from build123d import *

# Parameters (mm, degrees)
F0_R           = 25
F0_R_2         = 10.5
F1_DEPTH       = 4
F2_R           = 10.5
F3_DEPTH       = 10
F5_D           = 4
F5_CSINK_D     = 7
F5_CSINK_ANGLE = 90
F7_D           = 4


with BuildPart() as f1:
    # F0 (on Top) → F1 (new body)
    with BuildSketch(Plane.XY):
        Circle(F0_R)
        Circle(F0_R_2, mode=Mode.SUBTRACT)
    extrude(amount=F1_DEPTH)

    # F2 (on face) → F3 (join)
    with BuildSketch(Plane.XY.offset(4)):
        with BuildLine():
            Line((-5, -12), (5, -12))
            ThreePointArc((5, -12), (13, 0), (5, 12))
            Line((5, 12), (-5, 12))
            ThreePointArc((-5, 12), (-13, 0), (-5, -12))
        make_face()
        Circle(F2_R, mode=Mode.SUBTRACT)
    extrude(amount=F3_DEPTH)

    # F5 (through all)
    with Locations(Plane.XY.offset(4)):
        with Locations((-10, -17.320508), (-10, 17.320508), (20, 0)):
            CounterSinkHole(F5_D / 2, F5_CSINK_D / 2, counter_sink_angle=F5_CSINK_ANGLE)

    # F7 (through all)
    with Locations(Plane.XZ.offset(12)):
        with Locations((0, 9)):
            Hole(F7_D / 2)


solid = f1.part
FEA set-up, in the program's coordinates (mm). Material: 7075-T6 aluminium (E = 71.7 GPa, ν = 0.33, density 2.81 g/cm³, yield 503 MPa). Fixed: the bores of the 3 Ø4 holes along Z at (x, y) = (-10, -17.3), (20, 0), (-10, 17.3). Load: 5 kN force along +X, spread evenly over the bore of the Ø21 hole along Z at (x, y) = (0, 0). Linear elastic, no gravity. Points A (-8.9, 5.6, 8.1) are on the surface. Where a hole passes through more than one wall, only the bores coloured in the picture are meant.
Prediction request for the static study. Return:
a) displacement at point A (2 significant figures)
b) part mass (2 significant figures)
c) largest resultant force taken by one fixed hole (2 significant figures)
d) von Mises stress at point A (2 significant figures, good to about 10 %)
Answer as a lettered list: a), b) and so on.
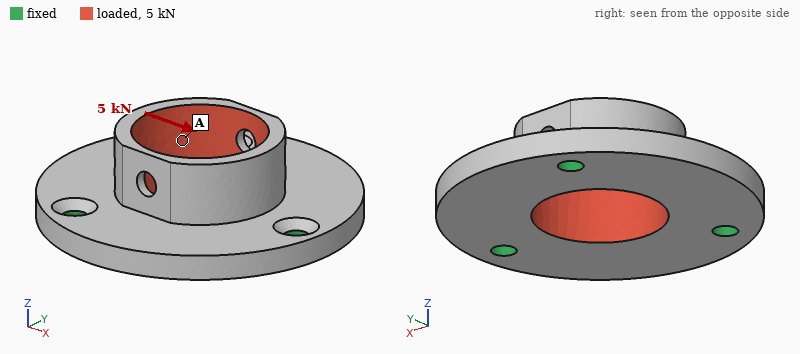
a) 32 µm
b) 22 g
c) 1.8 kN
d) 32 MPa
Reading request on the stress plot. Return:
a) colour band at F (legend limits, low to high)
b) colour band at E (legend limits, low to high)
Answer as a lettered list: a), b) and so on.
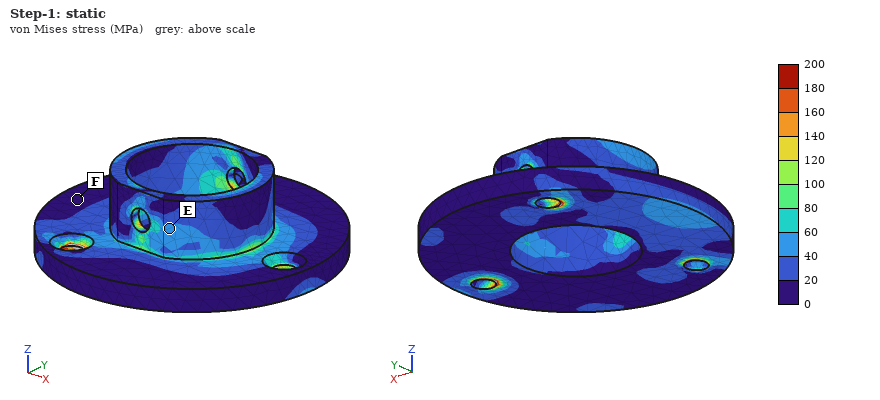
a) 0 to 20 MPa
b) 40 to 60 MPa
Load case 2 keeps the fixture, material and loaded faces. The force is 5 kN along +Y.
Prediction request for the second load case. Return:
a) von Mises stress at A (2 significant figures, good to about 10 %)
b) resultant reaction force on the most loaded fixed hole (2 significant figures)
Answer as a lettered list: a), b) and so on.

a) 45 MPa
b) 1.8 kN
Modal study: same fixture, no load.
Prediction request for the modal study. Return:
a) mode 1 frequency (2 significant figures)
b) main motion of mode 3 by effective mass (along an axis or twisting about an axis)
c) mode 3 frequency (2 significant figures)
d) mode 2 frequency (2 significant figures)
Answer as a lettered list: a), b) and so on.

a) 9500 Hz
b) along Z
c) 12 kHz
d) 9700 Hz
